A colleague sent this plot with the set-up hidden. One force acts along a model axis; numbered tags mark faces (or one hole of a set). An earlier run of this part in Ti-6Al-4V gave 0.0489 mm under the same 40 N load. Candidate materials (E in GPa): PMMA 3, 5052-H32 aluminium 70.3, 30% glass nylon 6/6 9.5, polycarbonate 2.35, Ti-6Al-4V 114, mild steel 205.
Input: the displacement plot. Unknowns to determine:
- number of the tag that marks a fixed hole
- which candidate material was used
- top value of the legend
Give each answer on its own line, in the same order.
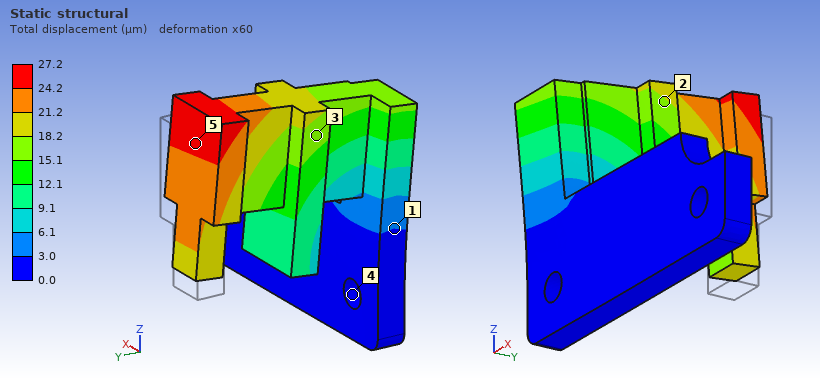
4
mild steel
27.2 µm
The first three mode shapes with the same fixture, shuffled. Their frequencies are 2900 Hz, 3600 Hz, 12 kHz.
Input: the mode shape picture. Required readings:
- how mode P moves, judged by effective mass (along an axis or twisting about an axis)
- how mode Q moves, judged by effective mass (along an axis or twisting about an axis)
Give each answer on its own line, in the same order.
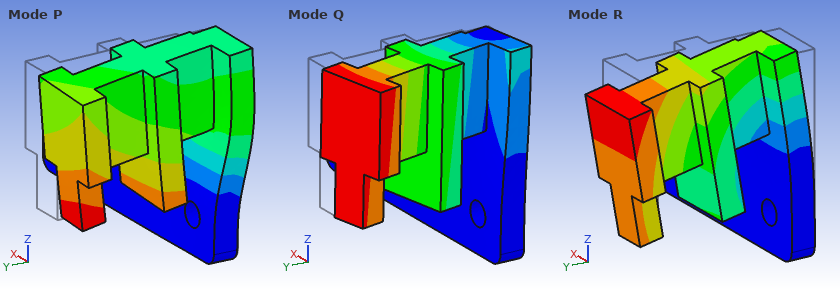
along Y
along X
